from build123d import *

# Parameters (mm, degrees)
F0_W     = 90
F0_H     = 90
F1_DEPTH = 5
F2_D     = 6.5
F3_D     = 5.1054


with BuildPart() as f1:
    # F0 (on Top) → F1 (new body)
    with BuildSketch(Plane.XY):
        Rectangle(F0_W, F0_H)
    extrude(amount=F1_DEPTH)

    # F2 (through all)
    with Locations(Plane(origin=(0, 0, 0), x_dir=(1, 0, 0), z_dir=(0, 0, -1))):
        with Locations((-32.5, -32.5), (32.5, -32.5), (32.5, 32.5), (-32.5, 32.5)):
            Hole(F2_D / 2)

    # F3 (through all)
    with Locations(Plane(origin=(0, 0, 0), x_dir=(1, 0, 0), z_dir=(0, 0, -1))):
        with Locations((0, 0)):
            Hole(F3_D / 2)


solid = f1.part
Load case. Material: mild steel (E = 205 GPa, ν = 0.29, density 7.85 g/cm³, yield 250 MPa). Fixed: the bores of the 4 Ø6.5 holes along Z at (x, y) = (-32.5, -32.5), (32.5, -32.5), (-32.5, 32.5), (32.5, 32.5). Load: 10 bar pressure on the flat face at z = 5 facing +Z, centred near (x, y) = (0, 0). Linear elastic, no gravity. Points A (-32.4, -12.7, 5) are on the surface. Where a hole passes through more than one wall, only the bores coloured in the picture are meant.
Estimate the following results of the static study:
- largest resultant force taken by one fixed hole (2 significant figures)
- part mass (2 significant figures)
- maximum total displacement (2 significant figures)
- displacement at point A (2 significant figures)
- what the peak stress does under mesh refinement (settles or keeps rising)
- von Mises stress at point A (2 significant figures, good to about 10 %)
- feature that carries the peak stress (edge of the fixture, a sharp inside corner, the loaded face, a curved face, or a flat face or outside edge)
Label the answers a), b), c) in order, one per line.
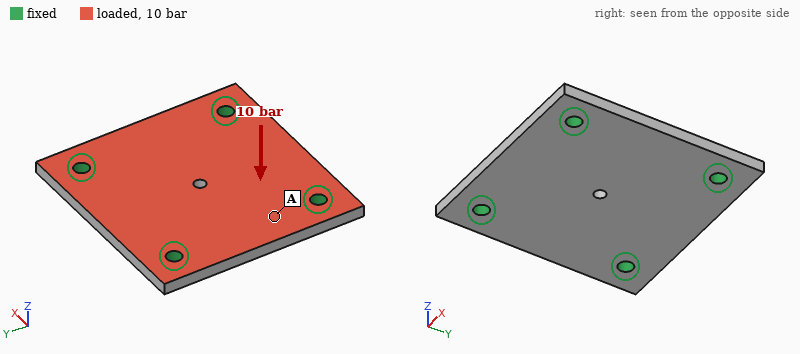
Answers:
a) 2.0 kN
b) 310 g
c) 49 µm
d) 20 µm
e) keeps rising
f) 33 MPa
g) edge of the fixture
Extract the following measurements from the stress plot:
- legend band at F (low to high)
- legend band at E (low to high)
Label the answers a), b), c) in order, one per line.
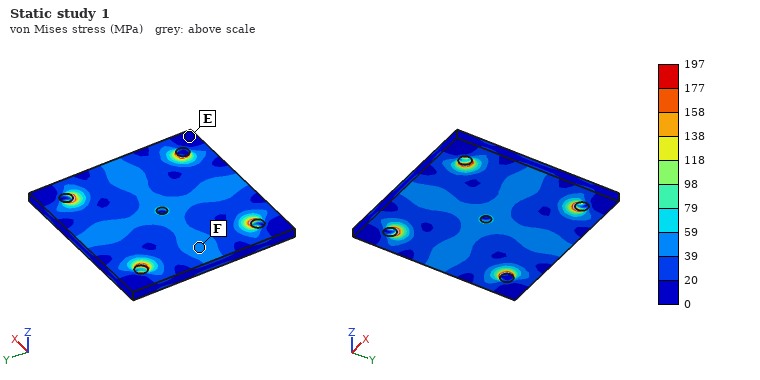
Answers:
a) 39 to 59 MPa
b) 0 to 20 MPa
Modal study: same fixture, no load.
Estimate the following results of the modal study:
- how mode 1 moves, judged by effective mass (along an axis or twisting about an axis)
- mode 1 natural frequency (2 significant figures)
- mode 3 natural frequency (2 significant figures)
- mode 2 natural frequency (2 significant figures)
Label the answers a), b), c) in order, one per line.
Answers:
a) along Z
b) 4500 Hz
c) 6800 Hz
d) 6800 Hz
